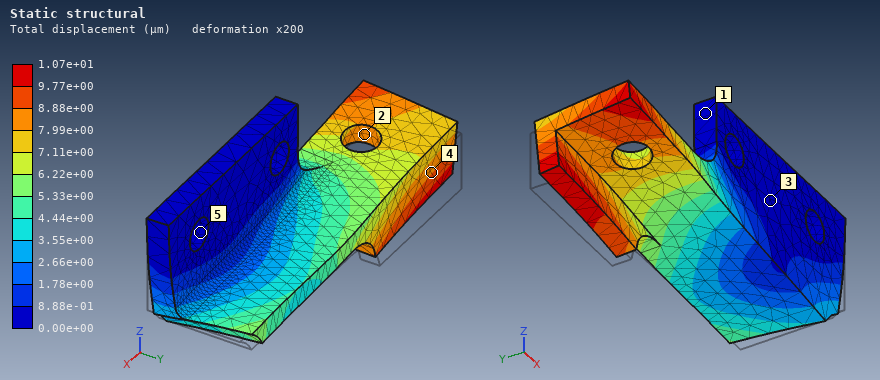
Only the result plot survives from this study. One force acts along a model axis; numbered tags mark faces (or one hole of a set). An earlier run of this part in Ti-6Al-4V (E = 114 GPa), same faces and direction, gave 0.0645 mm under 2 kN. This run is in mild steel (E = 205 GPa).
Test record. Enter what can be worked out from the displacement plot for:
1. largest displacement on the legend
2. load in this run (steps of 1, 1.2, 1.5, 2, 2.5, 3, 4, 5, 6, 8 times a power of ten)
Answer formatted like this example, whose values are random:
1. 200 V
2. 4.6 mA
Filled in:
1. 1.07e+01 µm
2. 600 N
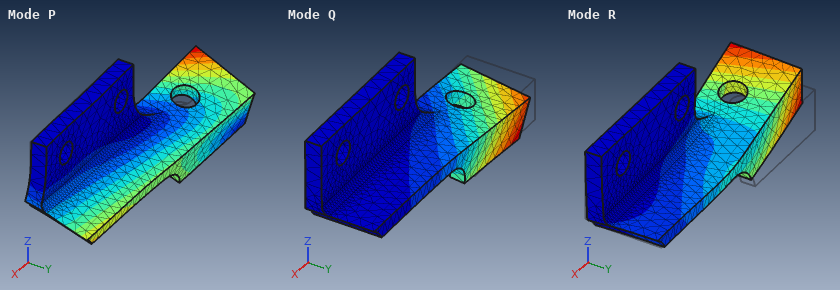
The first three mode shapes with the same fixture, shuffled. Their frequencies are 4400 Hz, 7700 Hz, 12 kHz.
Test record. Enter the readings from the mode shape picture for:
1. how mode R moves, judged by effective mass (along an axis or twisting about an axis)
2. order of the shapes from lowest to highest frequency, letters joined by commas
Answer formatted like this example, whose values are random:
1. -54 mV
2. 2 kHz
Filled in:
1. along Y
2. Q, R, P
